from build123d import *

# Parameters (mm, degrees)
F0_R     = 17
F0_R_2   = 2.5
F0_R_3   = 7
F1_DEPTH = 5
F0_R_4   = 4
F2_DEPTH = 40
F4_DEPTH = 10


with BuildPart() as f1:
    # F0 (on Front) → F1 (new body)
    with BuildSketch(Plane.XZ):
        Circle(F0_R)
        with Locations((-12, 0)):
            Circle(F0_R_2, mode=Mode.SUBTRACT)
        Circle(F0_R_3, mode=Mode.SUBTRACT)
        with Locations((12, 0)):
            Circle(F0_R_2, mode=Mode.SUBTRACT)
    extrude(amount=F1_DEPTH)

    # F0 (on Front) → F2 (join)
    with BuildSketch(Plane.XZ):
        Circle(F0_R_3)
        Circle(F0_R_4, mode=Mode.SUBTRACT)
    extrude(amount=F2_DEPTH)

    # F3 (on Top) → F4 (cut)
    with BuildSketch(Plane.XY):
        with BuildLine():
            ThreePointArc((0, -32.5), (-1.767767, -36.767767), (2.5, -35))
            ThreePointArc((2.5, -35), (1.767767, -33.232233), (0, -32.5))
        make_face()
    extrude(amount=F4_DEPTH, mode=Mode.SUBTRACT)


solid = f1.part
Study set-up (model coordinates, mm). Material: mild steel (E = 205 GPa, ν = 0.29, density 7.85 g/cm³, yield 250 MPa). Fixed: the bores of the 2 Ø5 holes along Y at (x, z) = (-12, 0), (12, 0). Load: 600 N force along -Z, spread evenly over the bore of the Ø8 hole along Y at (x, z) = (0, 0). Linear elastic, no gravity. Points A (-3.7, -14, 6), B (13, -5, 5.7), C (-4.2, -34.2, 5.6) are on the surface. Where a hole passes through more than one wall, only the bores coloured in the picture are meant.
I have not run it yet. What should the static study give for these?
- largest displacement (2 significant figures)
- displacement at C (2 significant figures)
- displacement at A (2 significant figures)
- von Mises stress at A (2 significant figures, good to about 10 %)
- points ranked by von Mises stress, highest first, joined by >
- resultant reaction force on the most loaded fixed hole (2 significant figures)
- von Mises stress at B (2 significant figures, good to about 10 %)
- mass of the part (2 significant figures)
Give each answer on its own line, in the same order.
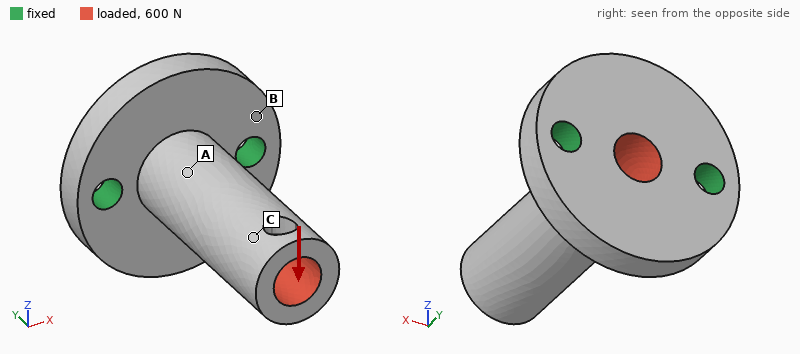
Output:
31 µm
26 µm
9.1 µm
17 MPa
B > A > C
300 N
26 MPa
60 g
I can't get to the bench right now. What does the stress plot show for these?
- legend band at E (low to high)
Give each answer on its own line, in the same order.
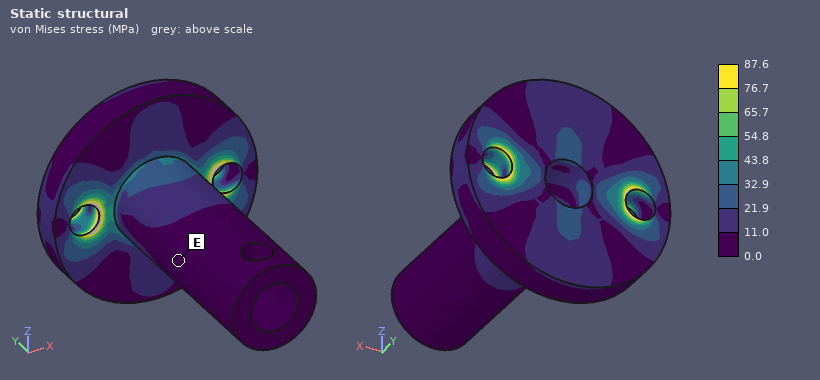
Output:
0.0 to 11.0 MPa
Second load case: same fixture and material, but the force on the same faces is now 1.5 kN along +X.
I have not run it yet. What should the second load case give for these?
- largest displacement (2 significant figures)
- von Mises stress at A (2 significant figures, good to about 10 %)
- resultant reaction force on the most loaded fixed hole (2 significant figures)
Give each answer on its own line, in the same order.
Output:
39 µm
33 MPa
1.6 kN
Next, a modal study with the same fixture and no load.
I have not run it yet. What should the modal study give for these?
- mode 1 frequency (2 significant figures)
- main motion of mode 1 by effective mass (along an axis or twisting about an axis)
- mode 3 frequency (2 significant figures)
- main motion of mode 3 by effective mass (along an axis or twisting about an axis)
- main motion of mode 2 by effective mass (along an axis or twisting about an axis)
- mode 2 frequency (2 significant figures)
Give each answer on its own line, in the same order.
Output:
4700 Hz
along Z
18 kHz
along Y
along X
6700 Hz
